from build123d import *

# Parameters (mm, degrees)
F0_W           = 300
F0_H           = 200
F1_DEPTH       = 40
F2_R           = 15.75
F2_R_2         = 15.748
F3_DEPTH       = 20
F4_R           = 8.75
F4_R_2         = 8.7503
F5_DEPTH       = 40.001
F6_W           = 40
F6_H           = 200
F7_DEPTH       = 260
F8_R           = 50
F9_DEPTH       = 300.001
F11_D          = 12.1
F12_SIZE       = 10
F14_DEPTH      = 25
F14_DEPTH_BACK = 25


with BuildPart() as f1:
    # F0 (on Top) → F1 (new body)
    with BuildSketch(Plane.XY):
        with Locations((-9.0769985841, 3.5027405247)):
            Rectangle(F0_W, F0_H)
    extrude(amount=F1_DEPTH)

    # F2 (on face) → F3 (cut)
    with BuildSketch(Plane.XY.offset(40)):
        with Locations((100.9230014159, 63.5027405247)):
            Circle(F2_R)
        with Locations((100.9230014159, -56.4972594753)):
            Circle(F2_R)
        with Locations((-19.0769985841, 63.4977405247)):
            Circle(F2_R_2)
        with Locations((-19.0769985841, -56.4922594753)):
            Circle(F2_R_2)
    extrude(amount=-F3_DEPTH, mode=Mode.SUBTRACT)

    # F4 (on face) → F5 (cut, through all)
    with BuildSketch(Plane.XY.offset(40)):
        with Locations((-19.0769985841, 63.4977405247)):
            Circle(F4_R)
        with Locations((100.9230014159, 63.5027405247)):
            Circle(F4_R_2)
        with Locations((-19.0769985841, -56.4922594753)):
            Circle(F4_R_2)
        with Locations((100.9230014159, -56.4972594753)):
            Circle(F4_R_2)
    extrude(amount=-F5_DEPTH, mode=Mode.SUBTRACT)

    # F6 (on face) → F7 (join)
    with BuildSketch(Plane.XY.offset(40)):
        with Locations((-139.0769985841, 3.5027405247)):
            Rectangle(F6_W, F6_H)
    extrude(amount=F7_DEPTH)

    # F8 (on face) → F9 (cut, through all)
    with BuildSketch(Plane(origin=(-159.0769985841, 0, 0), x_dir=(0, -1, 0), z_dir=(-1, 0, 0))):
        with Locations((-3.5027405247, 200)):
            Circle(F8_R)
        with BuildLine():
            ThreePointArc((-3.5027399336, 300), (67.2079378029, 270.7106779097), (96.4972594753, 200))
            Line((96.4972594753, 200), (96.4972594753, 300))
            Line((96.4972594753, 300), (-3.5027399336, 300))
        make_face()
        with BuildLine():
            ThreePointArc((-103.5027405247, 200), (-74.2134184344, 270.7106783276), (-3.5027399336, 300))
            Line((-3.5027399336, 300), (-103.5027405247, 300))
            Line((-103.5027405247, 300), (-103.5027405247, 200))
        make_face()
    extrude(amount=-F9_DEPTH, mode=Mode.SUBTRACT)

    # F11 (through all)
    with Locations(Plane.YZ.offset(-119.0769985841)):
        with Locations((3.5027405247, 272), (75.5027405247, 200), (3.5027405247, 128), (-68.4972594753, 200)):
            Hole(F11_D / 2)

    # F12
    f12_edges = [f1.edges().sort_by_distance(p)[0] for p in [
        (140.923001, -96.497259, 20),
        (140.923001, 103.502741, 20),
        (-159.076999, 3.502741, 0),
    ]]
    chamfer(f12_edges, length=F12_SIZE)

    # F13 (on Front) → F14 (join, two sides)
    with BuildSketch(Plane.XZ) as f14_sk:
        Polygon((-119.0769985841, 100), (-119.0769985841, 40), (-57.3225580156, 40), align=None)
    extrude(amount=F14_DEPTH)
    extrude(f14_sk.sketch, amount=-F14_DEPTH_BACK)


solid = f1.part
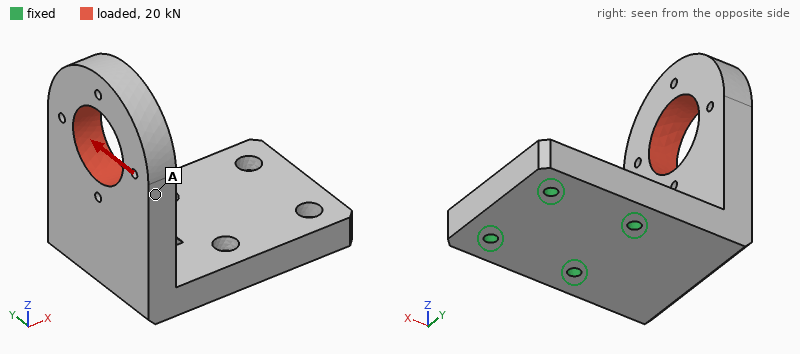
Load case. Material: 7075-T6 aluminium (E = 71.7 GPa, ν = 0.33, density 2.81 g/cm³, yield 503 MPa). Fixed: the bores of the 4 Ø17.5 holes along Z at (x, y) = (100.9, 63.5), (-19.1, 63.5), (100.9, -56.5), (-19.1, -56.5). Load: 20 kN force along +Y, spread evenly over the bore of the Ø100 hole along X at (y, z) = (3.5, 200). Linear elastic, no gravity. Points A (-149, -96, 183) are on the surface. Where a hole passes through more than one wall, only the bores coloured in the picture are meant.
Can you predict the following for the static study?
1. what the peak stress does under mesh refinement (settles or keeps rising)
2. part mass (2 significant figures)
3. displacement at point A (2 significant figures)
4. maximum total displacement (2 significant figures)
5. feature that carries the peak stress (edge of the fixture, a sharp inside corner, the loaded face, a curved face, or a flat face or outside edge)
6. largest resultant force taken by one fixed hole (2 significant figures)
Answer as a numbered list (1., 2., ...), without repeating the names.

1. keeps rising
2. 11 kg
3. 0.44 mm
4. 0.66 mm
5. edge of the fixture
6. 39 kN
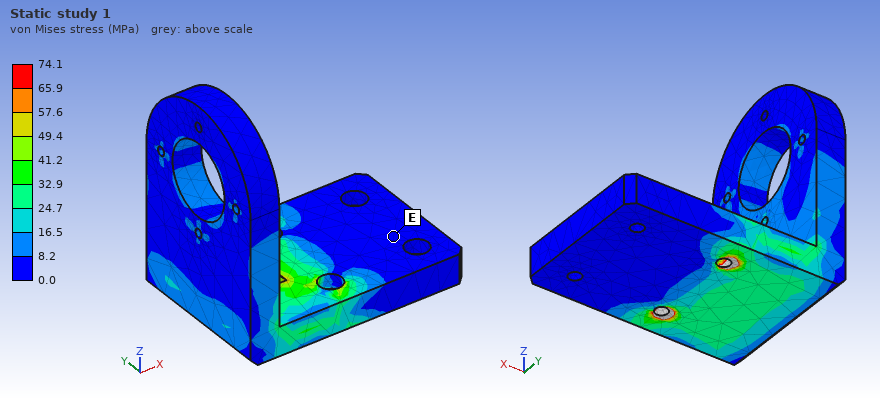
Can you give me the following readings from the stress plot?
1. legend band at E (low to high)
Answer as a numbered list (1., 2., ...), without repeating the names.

1. 0.0 to 8.2 MPa
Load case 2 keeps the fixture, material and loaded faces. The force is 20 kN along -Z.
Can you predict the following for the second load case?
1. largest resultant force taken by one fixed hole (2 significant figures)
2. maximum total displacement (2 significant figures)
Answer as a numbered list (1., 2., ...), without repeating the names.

1. 21 kN
2. 0.76 mm
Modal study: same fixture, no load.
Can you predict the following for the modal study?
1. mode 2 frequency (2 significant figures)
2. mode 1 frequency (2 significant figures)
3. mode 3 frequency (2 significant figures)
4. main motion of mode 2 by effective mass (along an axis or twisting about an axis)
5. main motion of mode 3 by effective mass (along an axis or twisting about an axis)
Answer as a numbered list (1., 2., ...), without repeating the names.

1. 570 Hz
2. 320 Hz
3. 980 Hz
4. along Y
5. along Z
